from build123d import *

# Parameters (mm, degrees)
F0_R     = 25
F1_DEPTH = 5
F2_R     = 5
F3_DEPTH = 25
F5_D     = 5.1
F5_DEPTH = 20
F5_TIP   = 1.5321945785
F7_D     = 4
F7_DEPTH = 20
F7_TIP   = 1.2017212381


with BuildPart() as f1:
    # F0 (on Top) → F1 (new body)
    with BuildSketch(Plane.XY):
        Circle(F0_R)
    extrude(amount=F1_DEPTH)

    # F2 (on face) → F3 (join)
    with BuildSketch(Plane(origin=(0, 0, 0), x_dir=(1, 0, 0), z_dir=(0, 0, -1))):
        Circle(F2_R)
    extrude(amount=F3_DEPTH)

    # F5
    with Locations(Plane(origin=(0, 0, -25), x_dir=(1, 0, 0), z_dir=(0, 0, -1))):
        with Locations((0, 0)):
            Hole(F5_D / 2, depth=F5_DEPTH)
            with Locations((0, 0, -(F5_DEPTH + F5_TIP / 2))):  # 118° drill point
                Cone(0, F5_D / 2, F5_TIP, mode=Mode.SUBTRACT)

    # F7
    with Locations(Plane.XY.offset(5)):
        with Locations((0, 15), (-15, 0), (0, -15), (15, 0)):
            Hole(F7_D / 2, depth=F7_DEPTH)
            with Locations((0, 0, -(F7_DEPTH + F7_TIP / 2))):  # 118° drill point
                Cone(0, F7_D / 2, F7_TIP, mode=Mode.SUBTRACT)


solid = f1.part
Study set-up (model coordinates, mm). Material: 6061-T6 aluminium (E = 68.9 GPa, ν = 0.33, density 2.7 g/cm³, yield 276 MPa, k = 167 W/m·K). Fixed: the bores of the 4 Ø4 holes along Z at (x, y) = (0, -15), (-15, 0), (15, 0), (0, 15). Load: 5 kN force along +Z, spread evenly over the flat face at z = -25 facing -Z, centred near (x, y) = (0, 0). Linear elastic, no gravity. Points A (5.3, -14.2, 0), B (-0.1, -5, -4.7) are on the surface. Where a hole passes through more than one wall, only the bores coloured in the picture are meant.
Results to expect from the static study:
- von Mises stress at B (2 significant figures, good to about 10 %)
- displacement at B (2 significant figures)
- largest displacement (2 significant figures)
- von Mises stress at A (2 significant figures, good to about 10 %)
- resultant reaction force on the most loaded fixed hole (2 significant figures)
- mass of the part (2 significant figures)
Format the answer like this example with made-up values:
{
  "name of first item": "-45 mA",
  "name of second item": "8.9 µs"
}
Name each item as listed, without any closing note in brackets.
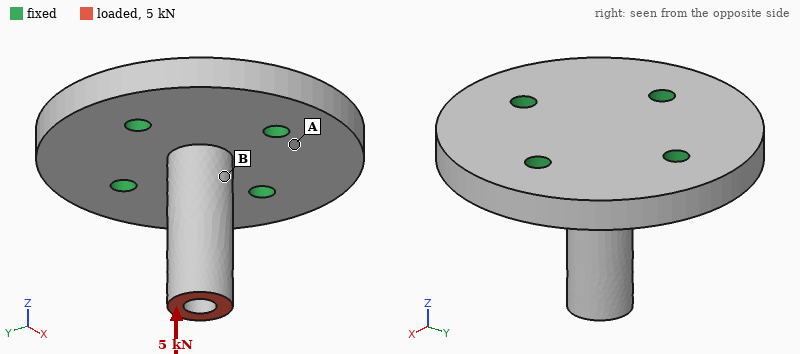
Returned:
{
  "von Mises stress at B": "75 MPa",
  "displacement at B": "31 µm",
  "largest displacement": "56 µm",
  "von Mises stress at A": "27 MPa",
  "resultant reaction force on the most loaded fixed hole": "1.3 kN",
  "mass of the part": "30 g"
}
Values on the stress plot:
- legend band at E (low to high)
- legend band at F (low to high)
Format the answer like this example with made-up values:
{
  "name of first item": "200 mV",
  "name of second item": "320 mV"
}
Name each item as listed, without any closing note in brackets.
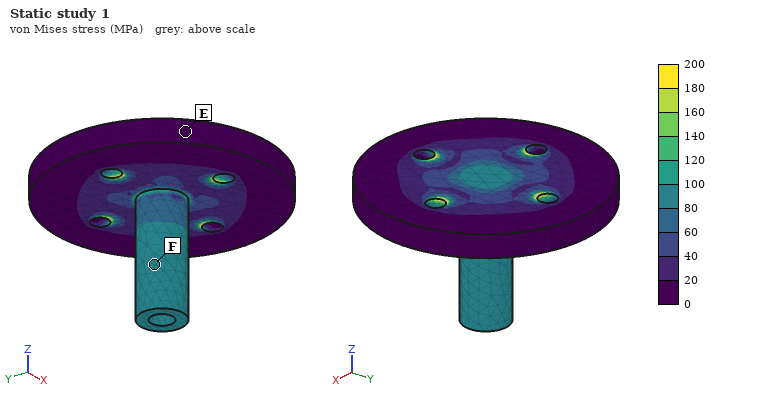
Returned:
{
  "legend band at E": "0 to 20 MPa",
  "legend band at F": "80 to 100 MPa"
}
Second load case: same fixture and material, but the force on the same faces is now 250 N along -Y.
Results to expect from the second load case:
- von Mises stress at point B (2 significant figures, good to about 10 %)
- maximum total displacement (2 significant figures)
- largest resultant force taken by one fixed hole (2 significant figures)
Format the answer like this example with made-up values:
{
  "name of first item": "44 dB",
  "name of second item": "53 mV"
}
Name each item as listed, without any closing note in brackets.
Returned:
{
  "von Mises stress at point B": "55 MPa",
  "maximum total displacement": "71 µm",
  "largest resultant force taken by one fixed hole": "280 N"
}
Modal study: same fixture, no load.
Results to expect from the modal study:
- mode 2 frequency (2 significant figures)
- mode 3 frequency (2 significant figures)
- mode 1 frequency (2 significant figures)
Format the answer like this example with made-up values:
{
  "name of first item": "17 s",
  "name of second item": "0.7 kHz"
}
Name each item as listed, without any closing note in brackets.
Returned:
{
  "mode 2 frequency": "8900 Hz",
  "mode 3 frequency": "20 kHz",
  "mode 1 frequency": "8900 Hz"
}
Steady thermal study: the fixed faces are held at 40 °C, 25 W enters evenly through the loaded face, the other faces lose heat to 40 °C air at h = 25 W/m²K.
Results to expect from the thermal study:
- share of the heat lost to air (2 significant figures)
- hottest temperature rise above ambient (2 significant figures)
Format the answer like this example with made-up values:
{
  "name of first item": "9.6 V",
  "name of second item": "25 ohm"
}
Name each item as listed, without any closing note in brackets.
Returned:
{
  "share of the heat lost to air": "5.0 %",
  "hottest temperature rise above ambient": "69 K"
}
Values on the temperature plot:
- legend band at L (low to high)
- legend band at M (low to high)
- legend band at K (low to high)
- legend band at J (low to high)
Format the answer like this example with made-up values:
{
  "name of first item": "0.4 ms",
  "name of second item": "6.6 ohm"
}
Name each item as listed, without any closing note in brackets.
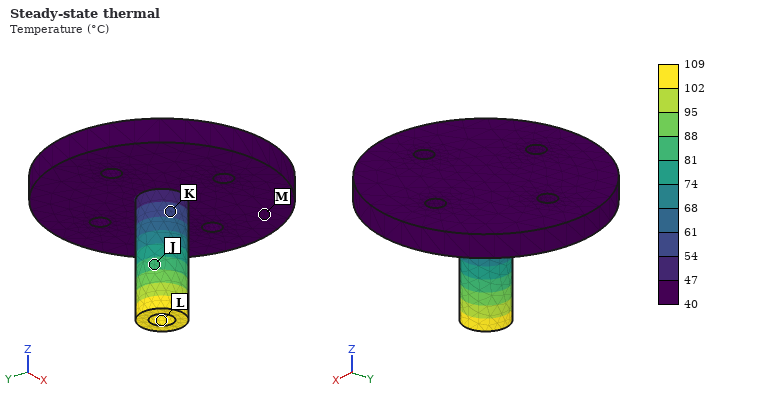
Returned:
{
  "legend band at L": "102 to 109 °C",
  "legend band at M": "40 to 47 °C",
  "legend band at K": "54 to 61 °C",
  "legend band at J": "81 to 88 °C"
}
